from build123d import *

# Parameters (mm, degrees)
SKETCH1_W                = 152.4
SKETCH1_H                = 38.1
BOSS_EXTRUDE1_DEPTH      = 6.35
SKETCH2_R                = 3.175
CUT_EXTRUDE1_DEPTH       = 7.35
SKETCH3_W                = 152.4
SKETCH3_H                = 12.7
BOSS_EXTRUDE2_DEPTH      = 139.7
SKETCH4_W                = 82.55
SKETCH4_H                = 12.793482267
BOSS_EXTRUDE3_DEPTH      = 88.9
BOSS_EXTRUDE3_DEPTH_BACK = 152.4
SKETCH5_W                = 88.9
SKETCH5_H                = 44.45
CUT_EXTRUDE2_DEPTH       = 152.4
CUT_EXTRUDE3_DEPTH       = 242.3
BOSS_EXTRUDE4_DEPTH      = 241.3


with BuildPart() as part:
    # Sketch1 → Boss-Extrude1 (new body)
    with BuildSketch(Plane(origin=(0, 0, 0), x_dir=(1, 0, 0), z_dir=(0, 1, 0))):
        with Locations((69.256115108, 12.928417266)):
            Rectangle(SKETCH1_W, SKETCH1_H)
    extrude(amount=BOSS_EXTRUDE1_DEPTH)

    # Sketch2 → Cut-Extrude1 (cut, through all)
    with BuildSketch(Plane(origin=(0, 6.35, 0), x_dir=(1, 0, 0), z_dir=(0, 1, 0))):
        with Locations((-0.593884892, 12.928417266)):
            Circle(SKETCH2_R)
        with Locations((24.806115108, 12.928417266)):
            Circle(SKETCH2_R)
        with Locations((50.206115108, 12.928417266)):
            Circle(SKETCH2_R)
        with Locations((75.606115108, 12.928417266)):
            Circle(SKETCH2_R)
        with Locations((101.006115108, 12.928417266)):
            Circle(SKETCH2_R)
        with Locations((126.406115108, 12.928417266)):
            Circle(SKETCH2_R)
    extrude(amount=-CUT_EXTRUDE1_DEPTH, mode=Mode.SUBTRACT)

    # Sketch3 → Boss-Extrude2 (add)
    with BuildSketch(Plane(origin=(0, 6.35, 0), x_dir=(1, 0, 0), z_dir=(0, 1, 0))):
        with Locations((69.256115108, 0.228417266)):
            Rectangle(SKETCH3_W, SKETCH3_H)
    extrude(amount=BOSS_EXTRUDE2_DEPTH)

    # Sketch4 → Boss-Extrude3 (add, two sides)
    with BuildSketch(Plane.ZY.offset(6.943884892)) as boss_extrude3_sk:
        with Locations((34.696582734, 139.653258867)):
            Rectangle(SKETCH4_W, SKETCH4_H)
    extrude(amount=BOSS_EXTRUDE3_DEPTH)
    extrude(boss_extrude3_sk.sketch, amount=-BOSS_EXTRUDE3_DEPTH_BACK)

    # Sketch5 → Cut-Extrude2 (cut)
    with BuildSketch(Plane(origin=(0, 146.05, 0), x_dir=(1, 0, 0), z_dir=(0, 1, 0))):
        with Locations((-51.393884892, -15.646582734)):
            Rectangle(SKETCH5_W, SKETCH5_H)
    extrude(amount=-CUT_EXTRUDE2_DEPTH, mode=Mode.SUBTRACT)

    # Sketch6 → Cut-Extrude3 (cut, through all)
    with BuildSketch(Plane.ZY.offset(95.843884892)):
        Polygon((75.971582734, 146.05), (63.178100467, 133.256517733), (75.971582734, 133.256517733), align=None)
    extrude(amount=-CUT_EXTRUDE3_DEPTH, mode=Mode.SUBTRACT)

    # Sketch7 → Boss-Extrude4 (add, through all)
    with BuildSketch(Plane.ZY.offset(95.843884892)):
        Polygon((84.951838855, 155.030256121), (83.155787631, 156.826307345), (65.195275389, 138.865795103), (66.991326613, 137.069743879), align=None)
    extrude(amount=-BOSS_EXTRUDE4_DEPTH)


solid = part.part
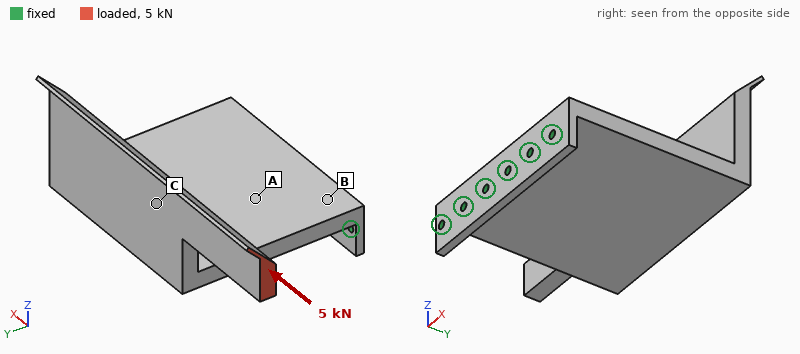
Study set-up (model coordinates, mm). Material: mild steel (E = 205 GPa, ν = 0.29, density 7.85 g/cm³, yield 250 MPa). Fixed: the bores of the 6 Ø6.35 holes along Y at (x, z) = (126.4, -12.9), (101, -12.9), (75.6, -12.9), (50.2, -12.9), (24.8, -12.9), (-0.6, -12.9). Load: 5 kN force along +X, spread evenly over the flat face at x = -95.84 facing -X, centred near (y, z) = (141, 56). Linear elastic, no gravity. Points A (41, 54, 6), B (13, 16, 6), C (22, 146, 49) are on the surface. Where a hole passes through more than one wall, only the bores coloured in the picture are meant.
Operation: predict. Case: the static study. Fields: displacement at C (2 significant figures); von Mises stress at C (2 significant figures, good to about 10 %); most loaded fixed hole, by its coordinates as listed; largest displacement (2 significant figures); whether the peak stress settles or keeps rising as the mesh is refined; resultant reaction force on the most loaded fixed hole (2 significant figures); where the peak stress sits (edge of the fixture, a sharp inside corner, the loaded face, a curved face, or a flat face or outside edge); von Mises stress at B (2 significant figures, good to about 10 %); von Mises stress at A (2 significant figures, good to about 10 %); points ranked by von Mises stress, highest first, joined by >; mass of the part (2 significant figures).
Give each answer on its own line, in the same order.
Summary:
0.23 mm
11 MPa
(126.4, -12.9)
0.63 mm
keeps rising
5.1 kN
edge of the fixture
41 MPa
55 MPa
A > B > C
3.7 kg
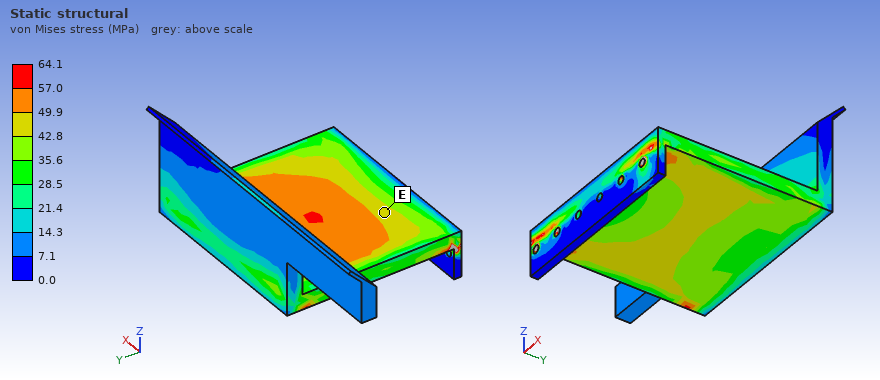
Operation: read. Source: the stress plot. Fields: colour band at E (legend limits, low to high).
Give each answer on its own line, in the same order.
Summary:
42.8 to 49.9 MPa
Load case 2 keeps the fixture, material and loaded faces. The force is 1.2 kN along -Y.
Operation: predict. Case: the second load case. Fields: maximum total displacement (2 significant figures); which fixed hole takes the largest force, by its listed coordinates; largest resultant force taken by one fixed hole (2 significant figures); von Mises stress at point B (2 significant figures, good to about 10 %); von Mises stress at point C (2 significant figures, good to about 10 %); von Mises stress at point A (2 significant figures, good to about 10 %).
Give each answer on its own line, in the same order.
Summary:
0.97 mm
(-0.6, -12.9)
1.3 kN
14 MPa
51 MPa
17 MPa
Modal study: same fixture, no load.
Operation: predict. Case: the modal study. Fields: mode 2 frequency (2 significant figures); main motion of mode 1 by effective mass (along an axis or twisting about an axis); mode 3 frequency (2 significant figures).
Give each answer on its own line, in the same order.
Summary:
430 Hz
along Z
650 Hz
